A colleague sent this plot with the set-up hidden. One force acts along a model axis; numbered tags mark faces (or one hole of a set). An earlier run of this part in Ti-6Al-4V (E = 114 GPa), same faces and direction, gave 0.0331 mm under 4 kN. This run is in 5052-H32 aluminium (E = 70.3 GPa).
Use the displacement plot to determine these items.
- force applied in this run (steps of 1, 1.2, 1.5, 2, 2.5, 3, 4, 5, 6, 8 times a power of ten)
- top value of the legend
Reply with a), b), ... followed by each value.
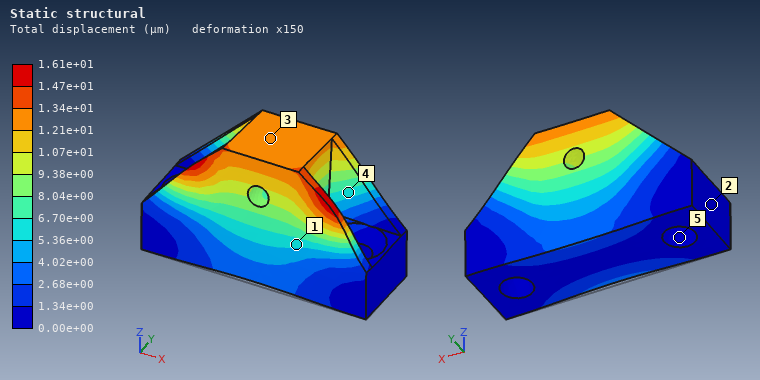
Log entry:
a) 1.2 kN
b) 1.61e+01 µm
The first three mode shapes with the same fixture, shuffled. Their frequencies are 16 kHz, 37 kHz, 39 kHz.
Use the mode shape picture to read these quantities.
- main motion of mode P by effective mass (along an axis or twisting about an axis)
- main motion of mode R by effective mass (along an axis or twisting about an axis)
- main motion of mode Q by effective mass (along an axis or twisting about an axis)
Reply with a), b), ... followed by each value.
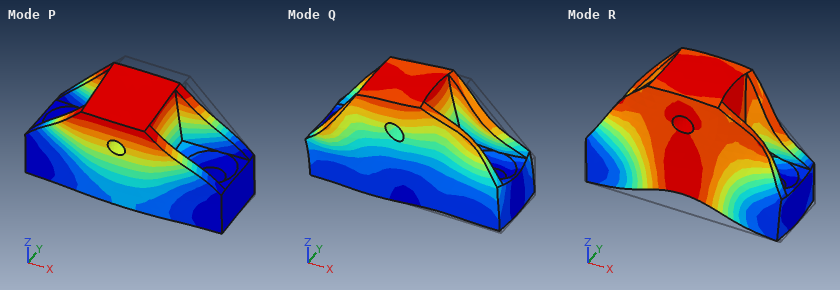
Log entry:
a) along Y
b) along Z
c) along X
